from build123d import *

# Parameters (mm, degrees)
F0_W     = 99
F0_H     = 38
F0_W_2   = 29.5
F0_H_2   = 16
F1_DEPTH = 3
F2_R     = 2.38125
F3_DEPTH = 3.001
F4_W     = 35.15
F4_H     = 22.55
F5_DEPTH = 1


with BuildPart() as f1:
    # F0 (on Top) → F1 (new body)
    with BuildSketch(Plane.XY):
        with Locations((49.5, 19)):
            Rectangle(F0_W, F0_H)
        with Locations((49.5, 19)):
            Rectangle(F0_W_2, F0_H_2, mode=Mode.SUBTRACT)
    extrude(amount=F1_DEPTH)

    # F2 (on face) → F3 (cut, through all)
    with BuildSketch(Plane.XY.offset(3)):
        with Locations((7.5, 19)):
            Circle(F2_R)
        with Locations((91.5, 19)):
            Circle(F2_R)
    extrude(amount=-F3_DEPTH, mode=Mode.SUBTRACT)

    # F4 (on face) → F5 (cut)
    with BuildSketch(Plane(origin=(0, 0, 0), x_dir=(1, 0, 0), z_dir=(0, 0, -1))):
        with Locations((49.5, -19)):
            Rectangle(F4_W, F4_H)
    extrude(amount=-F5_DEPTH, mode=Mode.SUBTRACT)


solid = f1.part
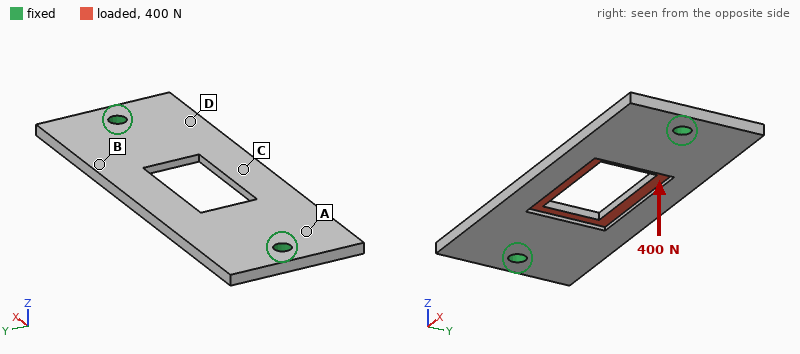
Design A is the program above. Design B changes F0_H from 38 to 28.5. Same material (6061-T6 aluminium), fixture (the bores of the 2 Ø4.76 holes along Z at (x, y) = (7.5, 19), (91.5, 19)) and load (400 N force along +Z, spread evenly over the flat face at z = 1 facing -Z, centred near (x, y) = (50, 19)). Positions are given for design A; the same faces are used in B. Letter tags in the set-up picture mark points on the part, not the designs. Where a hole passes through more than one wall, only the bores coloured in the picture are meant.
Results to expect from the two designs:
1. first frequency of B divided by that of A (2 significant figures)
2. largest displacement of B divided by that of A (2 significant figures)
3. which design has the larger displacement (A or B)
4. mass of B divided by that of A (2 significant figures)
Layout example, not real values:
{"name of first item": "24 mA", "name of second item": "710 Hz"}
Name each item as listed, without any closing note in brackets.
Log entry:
{"first frequency of B divided by that of A": "1.1", "largest displacement of B divided by that of A": "1.3", "which design has the larger displacement": "B", "mass of B divided by that of A": "0.70"}
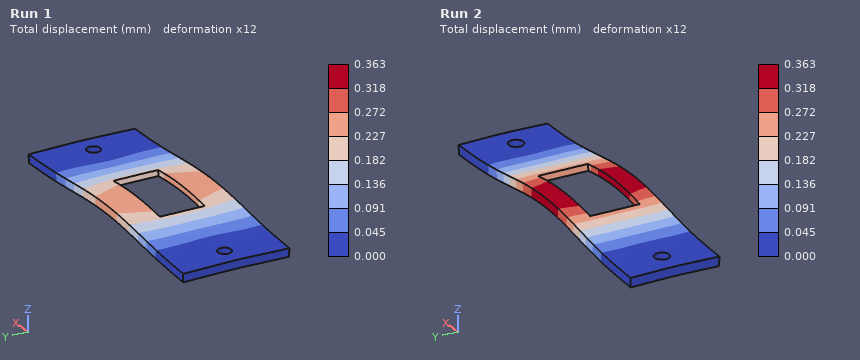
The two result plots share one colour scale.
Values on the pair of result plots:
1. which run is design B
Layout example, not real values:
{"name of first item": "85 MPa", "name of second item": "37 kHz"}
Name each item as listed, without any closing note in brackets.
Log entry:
{"which run is design B": "Run 2"}
